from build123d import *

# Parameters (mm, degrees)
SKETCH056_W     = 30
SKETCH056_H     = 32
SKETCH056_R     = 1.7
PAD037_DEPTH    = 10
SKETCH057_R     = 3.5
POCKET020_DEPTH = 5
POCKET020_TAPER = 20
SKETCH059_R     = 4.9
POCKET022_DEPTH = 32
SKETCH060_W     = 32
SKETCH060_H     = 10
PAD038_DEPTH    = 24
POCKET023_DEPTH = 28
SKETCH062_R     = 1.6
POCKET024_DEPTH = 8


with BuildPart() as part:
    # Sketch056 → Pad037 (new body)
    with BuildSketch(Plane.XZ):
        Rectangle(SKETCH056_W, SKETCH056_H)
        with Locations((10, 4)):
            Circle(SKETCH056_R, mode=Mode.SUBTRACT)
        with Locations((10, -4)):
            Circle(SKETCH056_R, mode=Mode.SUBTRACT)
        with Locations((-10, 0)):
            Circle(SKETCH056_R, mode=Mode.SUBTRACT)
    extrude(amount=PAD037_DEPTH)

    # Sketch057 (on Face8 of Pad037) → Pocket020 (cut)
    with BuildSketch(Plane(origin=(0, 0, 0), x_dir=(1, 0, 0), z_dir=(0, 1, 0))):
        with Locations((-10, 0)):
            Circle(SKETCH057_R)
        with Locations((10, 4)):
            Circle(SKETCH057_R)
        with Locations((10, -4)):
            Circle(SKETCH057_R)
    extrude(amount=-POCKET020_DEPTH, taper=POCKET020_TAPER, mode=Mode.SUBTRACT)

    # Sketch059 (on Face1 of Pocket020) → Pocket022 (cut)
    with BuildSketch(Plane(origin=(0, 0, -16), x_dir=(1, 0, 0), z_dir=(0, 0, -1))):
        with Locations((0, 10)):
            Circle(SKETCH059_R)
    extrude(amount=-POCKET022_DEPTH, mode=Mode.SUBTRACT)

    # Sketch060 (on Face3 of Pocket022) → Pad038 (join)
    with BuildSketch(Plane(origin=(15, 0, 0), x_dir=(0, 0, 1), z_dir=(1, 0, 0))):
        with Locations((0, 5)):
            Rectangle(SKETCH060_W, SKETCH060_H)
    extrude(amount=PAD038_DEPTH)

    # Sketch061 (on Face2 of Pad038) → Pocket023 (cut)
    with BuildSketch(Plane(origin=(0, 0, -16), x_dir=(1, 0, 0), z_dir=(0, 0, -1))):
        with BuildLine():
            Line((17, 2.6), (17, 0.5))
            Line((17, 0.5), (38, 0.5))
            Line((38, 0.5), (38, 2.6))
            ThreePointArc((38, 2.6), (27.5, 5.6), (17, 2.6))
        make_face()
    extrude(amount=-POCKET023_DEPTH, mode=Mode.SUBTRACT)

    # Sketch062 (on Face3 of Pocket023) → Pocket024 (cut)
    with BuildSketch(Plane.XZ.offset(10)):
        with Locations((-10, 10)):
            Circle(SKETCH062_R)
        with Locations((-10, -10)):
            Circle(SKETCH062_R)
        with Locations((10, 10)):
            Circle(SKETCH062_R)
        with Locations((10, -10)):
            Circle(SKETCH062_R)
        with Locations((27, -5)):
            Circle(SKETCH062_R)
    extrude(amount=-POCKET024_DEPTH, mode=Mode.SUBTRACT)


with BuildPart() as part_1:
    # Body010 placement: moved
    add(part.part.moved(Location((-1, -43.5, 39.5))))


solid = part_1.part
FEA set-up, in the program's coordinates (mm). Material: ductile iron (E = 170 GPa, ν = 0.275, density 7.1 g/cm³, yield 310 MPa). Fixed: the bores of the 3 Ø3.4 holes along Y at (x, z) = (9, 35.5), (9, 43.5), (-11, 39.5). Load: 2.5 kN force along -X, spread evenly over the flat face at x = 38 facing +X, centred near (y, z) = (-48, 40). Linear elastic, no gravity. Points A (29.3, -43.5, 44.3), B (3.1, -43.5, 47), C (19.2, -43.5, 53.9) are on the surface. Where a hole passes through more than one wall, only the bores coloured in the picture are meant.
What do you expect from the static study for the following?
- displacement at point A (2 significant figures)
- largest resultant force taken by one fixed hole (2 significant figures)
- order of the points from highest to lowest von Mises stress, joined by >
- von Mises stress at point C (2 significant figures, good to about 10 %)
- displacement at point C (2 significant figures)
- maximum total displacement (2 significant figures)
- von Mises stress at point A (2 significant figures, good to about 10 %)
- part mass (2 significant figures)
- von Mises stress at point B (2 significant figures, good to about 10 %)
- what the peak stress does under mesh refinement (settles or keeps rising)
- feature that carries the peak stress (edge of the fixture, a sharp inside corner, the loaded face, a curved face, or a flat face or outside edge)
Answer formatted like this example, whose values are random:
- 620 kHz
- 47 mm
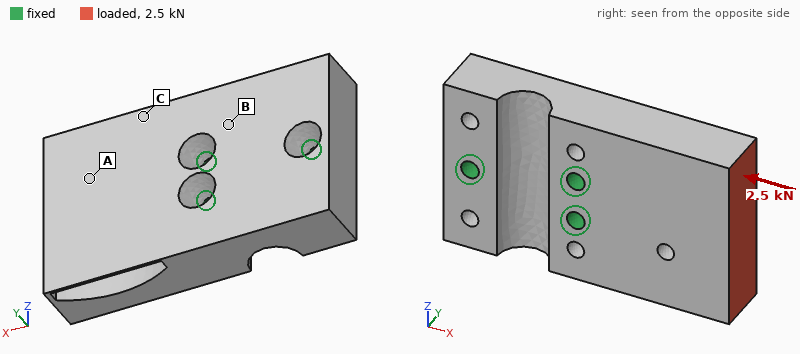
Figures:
- 7.3 µm
- 1.1 kN
- A > C > B
- 20 MPa
- 2.5 µm
- 12 µm
- 31 MPa
- 91 g
- 8.2 MPa
- keeps rising
- edge of the fixture
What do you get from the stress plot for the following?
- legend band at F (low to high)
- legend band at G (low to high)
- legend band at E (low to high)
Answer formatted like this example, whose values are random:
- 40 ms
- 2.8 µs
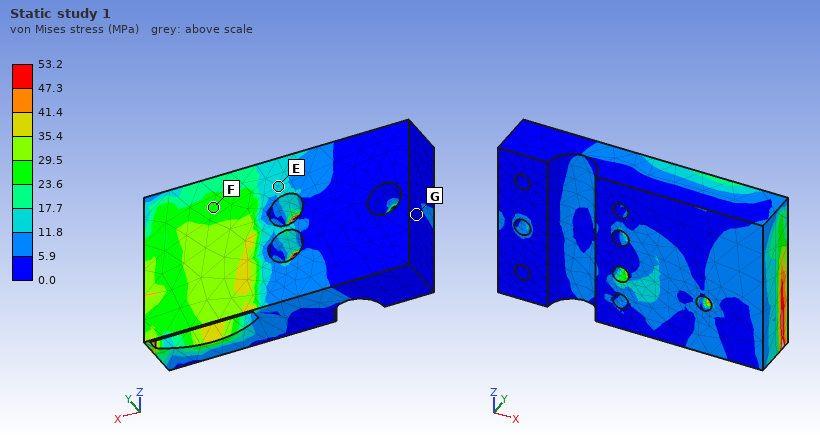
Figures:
- 23.6 to 29.5 MPa
- 0.0 to 5.9 MPa
- 11.8 to 17.7 MPa
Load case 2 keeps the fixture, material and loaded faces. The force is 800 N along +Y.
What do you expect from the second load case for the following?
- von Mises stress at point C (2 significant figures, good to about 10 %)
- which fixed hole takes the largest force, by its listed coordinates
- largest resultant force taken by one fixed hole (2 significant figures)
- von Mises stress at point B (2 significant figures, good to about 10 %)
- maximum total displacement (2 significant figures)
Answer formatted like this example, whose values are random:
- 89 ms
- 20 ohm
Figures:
- 56 MPa
- (-11, 39.5)
- 1.1 kN
- 30 MPa
- 47 µm
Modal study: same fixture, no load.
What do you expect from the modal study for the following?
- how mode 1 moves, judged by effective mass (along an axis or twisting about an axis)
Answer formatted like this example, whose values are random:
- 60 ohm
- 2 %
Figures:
- along Y
